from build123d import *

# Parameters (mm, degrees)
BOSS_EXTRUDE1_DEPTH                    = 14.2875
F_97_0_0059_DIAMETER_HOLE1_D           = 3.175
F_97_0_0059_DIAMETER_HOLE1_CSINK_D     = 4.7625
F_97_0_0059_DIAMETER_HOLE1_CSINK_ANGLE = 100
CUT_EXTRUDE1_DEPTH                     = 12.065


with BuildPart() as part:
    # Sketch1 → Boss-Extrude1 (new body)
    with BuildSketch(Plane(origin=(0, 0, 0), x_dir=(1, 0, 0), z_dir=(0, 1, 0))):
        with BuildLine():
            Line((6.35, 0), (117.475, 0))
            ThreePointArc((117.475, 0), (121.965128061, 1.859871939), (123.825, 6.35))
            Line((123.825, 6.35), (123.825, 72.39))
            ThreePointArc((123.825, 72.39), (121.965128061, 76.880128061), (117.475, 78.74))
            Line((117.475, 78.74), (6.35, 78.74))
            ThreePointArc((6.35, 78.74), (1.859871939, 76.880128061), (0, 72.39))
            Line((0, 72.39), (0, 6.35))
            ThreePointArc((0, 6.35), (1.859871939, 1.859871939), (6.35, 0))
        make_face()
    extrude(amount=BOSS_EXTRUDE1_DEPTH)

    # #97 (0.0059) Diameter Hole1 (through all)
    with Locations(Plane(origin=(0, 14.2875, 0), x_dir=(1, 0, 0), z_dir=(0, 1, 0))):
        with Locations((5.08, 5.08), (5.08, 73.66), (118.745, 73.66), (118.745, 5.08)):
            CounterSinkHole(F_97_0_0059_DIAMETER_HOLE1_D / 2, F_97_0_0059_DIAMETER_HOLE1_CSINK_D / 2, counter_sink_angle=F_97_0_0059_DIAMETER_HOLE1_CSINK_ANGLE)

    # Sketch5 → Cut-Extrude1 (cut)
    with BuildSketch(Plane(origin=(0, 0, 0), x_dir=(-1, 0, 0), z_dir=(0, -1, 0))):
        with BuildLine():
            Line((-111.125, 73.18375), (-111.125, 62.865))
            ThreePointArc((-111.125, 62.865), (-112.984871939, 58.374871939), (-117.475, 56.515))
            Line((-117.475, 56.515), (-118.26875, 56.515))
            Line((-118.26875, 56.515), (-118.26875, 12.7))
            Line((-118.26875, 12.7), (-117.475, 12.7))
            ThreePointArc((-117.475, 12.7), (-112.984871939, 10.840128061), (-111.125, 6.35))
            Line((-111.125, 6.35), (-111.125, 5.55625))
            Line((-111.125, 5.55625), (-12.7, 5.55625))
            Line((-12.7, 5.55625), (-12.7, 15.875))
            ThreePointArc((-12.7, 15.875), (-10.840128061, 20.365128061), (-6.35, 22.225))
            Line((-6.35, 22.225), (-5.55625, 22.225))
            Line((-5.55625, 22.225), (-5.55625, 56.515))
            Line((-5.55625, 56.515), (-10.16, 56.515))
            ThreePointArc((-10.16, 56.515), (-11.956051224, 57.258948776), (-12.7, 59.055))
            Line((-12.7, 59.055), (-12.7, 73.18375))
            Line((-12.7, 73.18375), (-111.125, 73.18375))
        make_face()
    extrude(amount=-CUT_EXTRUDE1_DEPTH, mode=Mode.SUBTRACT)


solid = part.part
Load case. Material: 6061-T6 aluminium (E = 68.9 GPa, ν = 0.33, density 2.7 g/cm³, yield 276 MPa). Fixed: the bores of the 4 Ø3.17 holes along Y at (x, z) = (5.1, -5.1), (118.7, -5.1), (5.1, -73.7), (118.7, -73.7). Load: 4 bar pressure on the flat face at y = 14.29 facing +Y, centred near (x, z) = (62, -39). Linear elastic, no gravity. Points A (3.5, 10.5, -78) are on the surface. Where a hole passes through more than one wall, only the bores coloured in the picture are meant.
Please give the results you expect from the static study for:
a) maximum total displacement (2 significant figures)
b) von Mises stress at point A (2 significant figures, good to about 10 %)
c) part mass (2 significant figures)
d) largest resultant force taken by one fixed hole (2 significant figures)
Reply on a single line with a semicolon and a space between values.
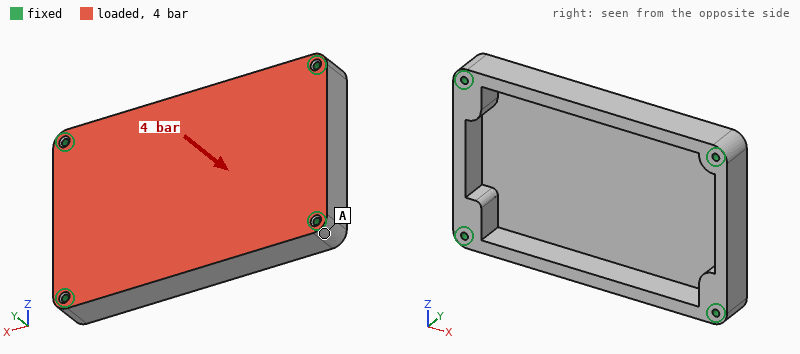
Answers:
0.47 mm; 12 MPa; 140 g; 1.1 kN
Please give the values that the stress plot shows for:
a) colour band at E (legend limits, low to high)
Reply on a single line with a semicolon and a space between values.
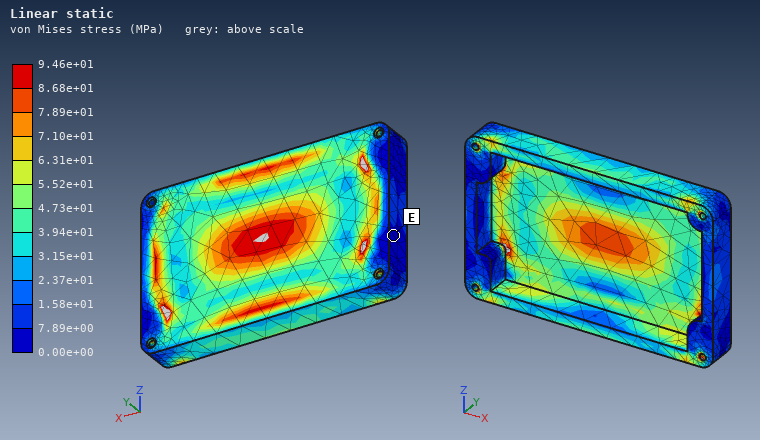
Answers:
0.00e+00 to 7.89e+00 MPa
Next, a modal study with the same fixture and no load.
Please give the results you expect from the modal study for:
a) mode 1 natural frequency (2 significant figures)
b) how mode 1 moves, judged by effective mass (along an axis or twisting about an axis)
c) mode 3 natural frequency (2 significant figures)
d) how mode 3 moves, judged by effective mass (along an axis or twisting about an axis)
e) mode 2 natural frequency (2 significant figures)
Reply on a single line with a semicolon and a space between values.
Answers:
2400 Hz; along Y; 4600 Hz; twisting about X; 4100 Hz
